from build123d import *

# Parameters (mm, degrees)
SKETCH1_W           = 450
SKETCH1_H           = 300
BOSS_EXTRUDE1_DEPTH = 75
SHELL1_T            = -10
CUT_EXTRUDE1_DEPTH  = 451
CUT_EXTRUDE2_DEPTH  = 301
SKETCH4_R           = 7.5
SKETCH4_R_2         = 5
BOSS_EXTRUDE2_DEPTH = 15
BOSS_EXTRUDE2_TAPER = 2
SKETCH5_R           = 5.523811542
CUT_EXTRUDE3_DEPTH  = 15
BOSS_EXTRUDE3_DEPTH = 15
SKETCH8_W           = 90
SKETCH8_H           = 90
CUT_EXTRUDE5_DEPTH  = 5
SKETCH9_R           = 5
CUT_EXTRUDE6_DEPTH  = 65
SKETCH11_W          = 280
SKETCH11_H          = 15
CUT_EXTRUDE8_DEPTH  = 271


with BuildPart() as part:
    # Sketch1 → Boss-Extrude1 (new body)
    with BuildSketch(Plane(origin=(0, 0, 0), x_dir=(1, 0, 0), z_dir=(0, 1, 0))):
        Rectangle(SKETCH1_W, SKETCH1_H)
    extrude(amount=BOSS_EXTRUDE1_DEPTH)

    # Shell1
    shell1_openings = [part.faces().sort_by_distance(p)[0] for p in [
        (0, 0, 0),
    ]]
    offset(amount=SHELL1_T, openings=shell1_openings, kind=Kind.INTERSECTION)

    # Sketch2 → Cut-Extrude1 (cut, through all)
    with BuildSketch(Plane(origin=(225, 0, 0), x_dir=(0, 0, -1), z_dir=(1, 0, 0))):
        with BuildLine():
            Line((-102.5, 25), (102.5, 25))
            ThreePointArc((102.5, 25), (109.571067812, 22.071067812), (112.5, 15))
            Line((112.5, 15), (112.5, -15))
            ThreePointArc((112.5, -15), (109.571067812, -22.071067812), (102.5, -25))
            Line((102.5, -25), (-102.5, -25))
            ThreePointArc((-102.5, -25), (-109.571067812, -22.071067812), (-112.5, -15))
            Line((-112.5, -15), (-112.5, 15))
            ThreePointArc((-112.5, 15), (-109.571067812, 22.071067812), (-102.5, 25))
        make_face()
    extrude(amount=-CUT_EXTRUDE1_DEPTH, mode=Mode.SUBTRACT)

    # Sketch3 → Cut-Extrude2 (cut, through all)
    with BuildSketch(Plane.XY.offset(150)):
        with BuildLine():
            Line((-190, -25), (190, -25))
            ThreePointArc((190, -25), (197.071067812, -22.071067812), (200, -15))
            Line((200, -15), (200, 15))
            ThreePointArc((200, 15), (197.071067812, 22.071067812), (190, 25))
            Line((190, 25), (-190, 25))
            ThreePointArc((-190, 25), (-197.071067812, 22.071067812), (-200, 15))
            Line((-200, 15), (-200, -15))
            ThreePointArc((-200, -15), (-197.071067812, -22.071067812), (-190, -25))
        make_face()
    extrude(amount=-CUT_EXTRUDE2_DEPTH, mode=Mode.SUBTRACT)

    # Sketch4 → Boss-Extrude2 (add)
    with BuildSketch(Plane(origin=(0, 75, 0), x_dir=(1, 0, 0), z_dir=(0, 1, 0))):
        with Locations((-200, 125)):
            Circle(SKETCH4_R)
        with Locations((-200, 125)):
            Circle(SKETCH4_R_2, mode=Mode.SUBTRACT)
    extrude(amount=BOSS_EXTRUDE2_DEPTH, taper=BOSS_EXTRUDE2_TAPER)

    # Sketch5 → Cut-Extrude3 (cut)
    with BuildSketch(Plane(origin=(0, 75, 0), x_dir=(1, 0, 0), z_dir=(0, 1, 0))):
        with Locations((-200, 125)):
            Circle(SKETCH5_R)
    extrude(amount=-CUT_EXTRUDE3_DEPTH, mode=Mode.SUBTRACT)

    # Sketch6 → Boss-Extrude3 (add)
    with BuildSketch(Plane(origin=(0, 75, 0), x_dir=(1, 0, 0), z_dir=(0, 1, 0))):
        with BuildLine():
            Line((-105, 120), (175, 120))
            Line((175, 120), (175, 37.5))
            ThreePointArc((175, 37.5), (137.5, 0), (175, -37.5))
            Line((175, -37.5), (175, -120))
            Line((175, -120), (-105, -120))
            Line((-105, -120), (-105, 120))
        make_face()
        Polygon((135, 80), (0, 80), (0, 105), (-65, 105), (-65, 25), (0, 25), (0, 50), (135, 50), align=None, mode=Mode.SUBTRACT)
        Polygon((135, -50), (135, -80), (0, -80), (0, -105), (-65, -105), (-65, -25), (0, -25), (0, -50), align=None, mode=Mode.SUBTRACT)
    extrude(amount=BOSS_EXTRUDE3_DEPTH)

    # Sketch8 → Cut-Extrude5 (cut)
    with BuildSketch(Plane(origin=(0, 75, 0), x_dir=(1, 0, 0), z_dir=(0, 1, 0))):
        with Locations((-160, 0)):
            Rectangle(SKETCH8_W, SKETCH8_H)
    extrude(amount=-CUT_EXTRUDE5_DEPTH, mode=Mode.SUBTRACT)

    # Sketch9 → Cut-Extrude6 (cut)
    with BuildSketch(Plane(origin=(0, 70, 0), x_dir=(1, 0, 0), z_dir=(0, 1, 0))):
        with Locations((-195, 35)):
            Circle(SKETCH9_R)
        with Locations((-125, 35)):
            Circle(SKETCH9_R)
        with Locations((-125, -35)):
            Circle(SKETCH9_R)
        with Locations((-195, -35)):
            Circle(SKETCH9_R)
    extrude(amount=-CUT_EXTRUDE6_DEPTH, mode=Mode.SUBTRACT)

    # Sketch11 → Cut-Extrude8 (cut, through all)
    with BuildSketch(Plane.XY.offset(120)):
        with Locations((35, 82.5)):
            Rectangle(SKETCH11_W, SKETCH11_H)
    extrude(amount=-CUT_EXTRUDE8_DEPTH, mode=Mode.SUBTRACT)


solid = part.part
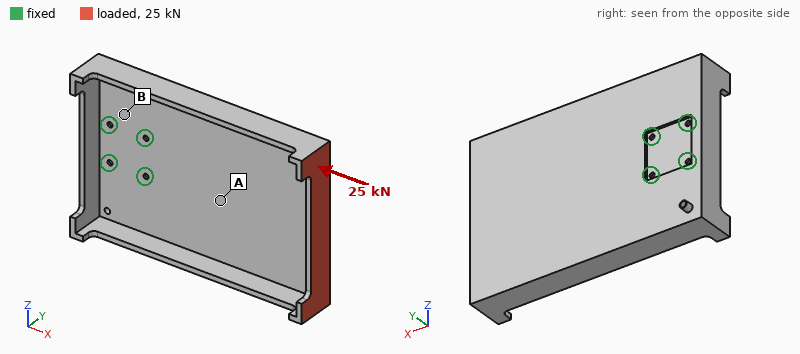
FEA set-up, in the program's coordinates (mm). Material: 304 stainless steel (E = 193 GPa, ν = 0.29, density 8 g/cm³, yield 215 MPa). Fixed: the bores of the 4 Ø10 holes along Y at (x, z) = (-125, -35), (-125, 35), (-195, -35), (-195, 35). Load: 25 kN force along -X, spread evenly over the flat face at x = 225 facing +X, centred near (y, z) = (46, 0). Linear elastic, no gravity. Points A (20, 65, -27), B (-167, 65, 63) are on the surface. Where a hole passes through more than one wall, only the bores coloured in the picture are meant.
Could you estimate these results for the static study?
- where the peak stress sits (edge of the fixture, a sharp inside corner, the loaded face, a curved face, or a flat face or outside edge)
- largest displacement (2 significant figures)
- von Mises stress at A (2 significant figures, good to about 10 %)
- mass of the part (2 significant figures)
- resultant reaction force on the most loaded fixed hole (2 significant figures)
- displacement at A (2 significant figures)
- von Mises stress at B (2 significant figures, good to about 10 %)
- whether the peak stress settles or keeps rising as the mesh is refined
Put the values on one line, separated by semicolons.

edge of the fixture; 1.6 mm; 15 MPa; 16 kg; 10 kN; 0.51 mm; 45 MPa; keeps rising
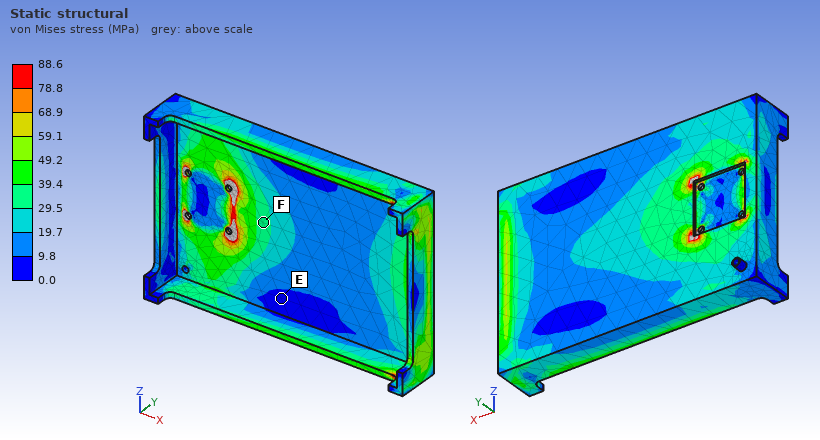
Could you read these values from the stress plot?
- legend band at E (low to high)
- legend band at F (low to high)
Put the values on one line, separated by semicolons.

0.0 to 9.8 MPa; 29.5 to 39.4 MPa
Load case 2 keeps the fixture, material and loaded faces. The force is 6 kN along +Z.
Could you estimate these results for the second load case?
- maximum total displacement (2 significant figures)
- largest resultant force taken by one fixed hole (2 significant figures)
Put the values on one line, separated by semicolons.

0.75 mm; 13 kN
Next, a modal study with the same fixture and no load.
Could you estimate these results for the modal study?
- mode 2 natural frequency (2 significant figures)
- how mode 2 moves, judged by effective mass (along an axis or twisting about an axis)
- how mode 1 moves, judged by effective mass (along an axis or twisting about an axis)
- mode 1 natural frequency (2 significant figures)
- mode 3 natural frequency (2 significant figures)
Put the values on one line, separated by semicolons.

120 Hz; twisting about X; along Y; 72 Hz; 460 Hz
